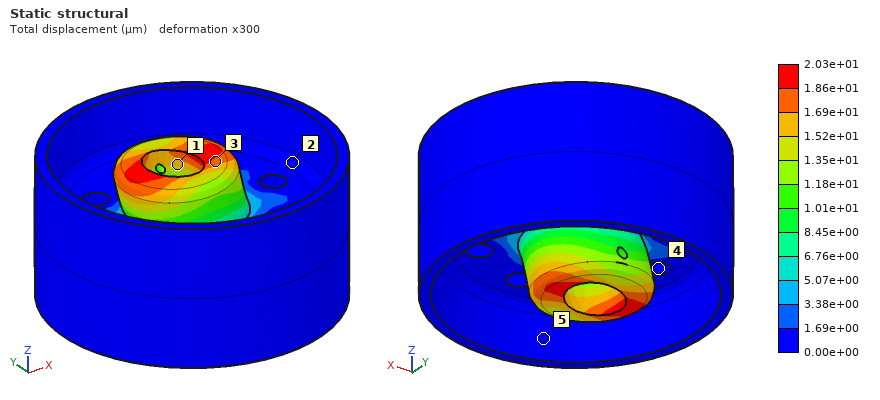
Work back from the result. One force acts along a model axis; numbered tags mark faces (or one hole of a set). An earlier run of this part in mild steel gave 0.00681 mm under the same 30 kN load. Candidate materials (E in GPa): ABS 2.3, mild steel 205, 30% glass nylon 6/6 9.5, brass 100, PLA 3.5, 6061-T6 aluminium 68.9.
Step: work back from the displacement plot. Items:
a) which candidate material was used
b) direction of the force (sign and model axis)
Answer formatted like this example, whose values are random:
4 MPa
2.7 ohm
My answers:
6061-T6 aluminium
-X
